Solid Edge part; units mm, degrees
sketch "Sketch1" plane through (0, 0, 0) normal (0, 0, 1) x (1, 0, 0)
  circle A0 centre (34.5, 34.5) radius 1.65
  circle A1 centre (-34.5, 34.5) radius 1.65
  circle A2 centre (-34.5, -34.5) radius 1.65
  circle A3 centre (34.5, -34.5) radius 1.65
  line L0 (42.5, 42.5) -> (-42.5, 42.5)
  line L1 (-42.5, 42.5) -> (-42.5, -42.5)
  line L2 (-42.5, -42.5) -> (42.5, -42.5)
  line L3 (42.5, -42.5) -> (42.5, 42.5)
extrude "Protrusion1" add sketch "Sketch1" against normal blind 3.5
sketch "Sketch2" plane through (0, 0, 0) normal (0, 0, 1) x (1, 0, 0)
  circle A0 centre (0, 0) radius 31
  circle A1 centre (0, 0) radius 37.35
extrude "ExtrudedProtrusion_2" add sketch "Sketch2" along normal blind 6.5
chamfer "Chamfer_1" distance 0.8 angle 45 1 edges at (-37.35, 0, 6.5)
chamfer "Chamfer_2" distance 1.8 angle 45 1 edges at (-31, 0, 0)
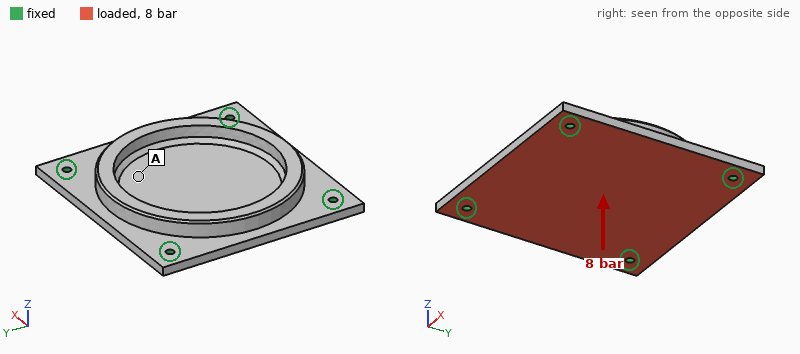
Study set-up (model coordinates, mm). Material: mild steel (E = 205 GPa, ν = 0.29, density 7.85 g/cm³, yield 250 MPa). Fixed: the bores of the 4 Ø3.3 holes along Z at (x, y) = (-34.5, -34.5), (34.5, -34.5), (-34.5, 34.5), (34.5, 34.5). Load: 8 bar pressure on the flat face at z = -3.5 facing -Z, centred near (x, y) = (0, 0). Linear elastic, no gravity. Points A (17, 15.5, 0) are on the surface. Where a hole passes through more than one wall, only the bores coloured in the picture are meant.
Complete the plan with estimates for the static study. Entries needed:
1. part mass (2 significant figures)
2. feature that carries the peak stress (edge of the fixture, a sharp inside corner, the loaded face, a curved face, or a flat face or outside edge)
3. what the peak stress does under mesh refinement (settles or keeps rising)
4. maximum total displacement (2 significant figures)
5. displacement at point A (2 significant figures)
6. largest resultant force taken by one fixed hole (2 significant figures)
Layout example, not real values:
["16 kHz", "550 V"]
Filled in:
["270 g", "edge of the fixture", "keeps rising", "73 µm", "51 µm", "1.6 kN"]
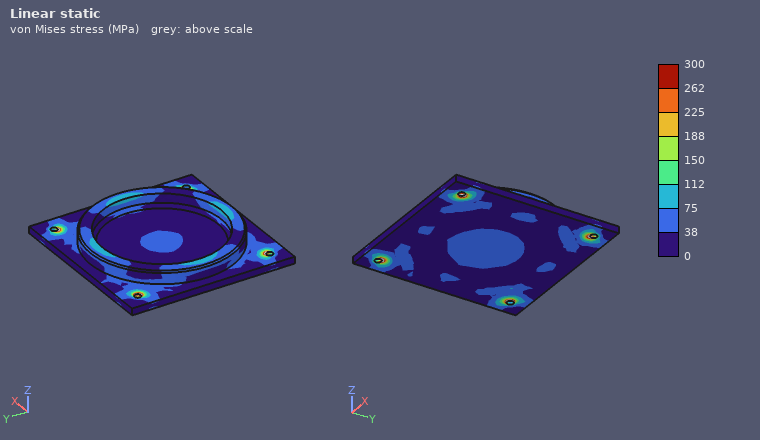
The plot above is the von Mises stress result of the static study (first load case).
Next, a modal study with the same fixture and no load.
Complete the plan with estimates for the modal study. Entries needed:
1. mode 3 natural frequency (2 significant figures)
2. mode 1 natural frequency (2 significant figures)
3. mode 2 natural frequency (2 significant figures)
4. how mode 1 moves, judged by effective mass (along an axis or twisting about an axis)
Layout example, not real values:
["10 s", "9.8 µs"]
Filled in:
["5100 Hz", "3500 Hz", "5100 Hz", "along Z"]
